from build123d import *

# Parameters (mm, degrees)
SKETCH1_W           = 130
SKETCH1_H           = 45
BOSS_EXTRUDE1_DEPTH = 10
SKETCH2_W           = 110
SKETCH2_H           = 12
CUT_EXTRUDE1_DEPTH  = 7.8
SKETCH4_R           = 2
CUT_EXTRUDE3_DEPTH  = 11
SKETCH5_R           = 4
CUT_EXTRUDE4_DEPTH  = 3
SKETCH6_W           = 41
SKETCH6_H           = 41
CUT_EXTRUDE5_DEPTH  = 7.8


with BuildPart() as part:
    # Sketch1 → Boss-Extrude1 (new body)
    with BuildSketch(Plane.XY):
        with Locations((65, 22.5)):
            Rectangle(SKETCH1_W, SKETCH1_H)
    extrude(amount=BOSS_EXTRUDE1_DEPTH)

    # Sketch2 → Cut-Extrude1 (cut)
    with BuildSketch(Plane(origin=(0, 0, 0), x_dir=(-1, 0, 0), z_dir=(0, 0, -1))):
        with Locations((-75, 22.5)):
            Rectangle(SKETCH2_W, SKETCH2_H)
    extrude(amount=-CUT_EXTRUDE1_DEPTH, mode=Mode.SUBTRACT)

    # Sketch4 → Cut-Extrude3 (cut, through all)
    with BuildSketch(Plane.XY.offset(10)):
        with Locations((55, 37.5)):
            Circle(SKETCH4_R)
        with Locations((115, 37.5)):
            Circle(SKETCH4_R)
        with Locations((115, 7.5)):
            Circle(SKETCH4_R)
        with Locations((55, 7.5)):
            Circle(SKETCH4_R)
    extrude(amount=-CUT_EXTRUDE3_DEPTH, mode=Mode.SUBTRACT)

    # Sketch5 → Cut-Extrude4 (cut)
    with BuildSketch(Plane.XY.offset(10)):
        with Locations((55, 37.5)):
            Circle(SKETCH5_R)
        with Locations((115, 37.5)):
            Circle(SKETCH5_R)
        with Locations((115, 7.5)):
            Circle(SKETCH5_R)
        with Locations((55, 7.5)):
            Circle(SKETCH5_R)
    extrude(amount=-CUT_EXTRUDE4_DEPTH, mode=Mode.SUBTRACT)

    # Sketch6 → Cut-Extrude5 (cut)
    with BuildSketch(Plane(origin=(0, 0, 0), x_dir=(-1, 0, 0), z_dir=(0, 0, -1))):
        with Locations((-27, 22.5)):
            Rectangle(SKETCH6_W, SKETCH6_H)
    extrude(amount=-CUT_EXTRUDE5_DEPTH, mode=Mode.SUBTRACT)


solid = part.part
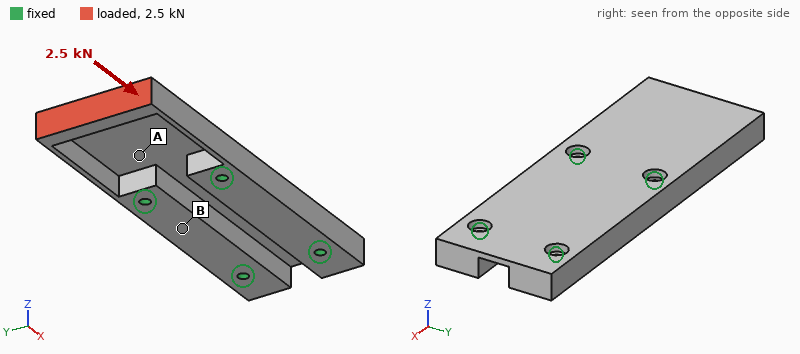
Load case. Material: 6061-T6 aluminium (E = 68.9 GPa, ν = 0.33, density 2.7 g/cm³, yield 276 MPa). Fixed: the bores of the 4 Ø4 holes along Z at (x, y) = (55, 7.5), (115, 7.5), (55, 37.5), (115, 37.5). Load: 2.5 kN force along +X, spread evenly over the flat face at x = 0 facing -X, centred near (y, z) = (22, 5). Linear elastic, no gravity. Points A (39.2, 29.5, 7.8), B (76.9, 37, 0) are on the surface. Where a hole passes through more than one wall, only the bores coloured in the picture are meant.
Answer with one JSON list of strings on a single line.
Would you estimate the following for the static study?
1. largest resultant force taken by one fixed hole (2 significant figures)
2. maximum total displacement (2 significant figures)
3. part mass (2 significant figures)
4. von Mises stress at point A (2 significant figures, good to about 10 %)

["1.1 kN", "0.21 mm", "99 g", "22 MPa"]
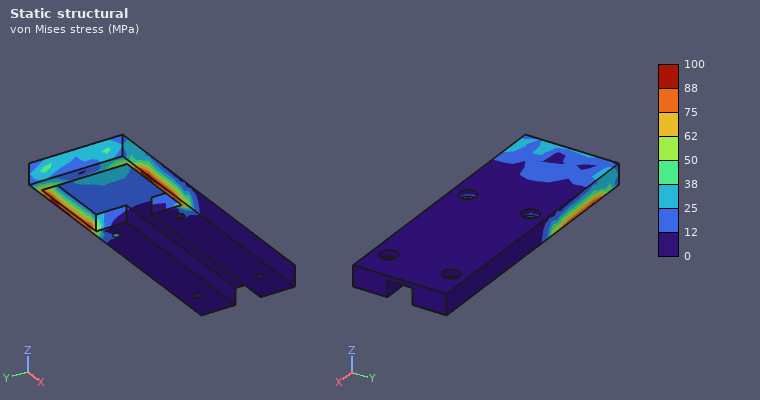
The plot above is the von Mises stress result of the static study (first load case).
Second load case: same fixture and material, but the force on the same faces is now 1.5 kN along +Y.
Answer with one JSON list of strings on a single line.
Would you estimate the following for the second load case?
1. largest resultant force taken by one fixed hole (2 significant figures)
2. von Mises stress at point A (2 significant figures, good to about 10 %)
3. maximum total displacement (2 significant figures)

["2.1 kN", "58 MPa", "0.31 mm"]
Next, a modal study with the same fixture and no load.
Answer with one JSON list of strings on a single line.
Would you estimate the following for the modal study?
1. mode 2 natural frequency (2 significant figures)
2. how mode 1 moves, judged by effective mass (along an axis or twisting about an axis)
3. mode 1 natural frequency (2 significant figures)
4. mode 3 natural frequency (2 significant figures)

["2800 Hz", "along Z", "1600 Hz", "6800 Hz"]
